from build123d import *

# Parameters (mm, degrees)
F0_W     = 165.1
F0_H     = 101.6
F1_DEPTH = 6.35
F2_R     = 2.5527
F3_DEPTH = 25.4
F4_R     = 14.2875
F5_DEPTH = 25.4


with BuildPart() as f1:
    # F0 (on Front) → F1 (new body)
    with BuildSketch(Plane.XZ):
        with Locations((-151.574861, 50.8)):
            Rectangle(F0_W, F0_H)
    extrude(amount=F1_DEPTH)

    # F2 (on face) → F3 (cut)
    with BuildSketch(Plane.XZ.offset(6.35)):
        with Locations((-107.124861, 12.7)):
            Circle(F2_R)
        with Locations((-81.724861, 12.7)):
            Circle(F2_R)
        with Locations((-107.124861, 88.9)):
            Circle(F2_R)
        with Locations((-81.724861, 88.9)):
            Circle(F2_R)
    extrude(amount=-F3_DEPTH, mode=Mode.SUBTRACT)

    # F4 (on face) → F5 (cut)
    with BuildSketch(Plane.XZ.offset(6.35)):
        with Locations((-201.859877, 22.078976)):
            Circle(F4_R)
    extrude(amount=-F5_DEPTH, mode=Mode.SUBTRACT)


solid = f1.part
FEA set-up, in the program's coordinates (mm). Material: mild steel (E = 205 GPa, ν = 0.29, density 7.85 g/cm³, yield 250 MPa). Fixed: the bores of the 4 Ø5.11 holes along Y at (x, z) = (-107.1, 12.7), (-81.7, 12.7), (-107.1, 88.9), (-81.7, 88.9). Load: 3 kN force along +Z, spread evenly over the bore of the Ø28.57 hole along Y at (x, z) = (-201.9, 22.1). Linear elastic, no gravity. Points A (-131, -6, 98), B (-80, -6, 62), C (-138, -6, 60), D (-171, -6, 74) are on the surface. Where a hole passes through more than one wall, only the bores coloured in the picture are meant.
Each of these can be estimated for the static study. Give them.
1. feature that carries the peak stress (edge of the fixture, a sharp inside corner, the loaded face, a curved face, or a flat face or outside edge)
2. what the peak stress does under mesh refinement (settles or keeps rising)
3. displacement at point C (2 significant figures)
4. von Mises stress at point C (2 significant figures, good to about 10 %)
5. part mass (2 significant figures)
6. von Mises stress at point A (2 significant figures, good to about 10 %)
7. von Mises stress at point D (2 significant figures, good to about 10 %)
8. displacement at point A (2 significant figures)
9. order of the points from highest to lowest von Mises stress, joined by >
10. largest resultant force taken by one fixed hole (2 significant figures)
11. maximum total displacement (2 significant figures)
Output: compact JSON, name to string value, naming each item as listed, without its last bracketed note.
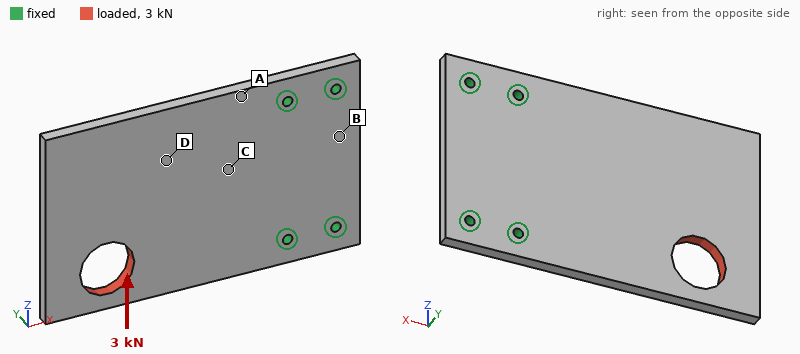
{"feature that carries the peak stress": "edge of the fixture", "what the peak stress does under mesh refinement": "keeps rising", "displacement at point C": "4.0 µm", "von Mises stress at point C": "11 MPa", "part mass": "800 g", "von Mises stress at point A": "17 MPa", "von Mises stress at point D": "8.8 MPa", "displacement at point A": "4.9 µm", "order of the points from highest to lowest von Mises stress, joined by >": "A > C > D > B", "largest resultant force taken by one fixed hole": "3.3 kN", "maximum total displacement": "23 µm"}
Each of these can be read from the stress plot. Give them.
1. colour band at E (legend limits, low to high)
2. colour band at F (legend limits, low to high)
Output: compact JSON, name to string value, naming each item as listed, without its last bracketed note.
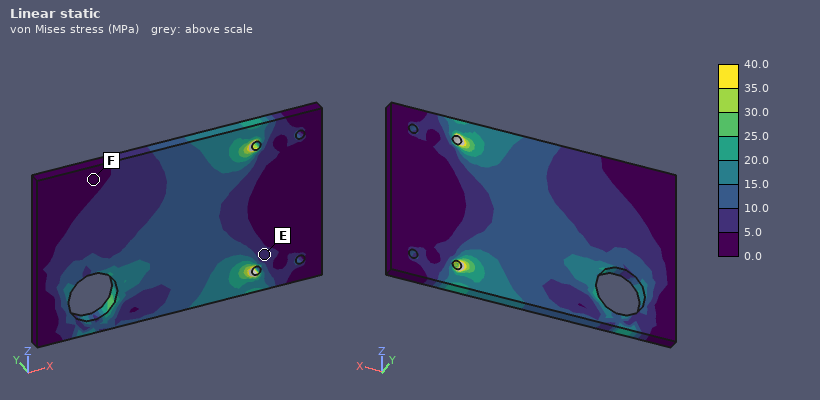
{"colour band at E": "5.0 to 10.0 MPa", "colour band at F": "0.0 to 5.0 MPa"}
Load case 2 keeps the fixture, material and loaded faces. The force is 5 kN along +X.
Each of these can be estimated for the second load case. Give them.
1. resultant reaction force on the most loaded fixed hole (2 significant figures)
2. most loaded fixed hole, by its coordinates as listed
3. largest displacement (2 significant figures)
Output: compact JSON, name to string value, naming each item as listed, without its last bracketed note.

{"resultant reaction force on the most loaded fixed hole": "3.3 kN", "most loaded fixed hole, by its coordinates as listed": "(-107.1, 12.7)", "largest displacement": "17 µm"}
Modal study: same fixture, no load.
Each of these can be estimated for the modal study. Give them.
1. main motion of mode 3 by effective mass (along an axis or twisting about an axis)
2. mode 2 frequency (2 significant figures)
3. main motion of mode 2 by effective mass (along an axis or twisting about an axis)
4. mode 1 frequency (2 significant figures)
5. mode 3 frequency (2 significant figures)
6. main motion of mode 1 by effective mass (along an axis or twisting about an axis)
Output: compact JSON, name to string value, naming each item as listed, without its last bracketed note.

{"main motion of mode 3 by effective mass": "along Y", "mode 2 frequency": "970 Hz", "main motion of mode 2 by effective mass": "twisting about X", "mode 1 frequency": "320 Hz", "mode 3 frequency": "1800 Hz", "main motion of mode 1 by effective mass": "along Y"}
